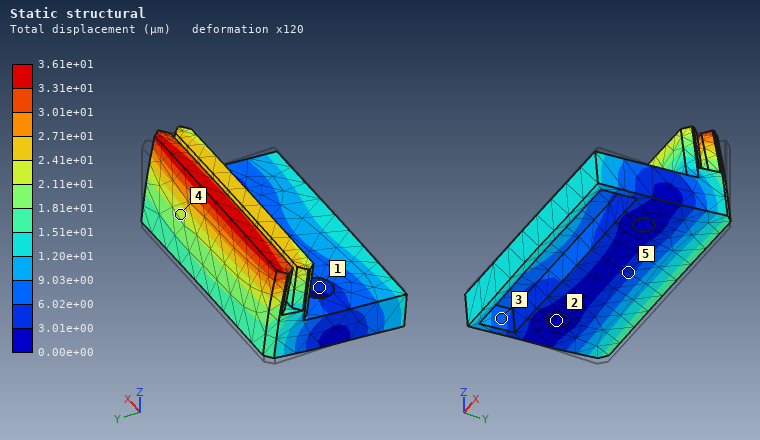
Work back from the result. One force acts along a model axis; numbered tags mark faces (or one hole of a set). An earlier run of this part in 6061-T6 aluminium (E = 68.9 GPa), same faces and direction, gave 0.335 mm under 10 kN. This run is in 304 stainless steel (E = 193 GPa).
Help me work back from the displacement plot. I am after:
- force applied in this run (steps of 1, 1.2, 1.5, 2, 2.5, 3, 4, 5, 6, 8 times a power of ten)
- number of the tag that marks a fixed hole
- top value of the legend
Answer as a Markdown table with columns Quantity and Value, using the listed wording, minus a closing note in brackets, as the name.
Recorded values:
| Quantity | Value |
|---|---|
| force applied in this run | 3 kN |
| number of the tag that marks a fixed hole | 2 |
| top value of the legend | 3.61e+01 µm |
